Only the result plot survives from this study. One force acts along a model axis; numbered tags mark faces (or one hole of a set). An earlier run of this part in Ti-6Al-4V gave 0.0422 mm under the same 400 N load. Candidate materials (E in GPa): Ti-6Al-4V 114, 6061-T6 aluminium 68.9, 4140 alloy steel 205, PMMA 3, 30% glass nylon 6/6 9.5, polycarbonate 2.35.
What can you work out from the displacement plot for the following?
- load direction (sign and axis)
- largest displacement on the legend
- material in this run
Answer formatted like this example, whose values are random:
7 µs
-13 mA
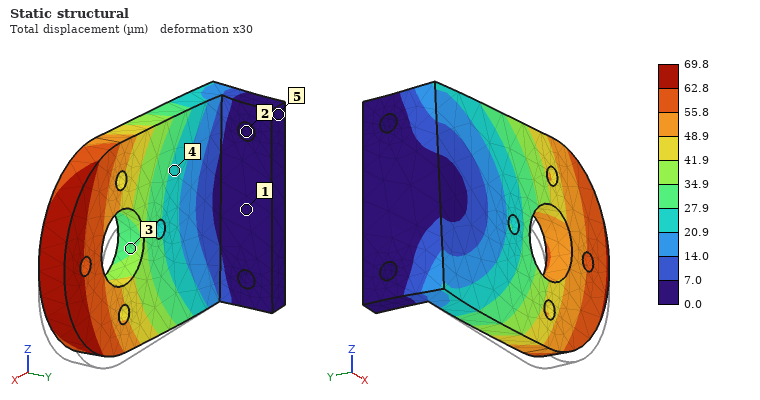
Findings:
+Z
69.8 µm
6061-T6 aluminium
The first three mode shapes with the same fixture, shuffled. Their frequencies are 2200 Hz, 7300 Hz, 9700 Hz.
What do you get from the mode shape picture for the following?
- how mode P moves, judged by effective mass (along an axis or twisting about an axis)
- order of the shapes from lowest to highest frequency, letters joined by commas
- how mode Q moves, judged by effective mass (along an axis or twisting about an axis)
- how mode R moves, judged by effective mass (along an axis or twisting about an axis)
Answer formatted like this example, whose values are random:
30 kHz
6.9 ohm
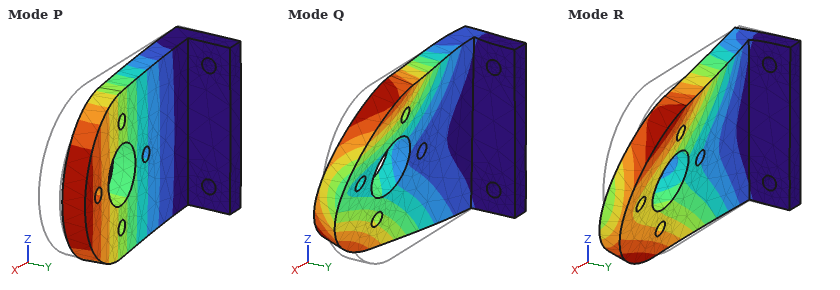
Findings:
along Y
P, R, Q
along Z
along Z
